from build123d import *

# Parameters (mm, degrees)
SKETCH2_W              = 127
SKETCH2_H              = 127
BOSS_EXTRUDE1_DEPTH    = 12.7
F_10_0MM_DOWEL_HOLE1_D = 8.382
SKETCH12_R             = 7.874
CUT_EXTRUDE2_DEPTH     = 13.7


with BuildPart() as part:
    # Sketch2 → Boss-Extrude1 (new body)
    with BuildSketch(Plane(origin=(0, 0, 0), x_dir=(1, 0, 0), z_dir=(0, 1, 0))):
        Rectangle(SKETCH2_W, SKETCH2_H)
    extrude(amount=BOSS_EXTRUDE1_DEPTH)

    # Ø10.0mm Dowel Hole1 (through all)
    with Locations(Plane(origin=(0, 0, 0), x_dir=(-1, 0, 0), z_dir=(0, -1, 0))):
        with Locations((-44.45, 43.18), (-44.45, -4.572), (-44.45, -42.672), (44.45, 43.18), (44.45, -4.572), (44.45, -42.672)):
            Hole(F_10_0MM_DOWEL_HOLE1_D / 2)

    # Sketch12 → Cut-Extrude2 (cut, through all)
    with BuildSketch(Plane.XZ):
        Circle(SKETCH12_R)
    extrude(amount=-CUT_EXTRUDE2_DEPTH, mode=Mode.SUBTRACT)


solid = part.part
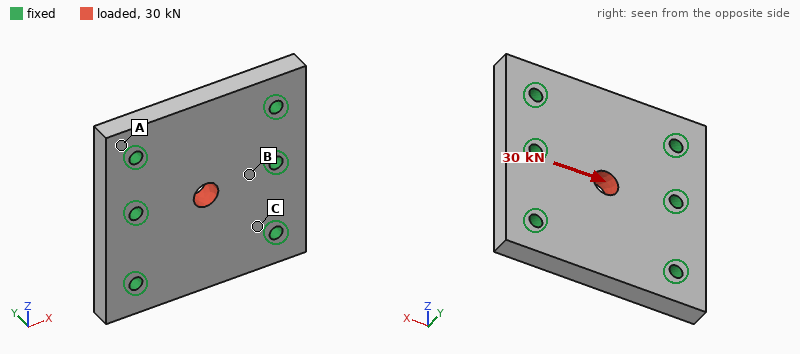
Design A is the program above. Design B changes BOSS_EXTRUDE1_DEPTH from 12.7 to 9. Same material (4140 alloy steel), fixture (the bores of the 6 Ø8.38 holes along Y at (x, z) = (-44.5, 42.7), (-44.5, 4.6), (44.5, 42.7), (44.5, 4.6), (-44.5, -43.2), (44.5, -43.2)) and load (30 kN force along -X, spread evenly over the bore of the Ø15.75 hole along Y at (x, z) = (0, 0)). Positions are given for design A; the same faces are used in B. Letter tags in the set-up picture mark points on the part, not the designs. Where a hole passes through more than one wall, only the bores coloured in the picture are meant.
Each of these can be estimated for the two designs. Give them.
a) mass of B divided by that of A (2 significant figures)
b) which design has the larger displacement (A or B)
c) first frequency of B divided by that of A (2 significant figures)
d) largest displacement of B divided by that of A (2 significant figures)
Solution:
0.71
B
0.77
1.4
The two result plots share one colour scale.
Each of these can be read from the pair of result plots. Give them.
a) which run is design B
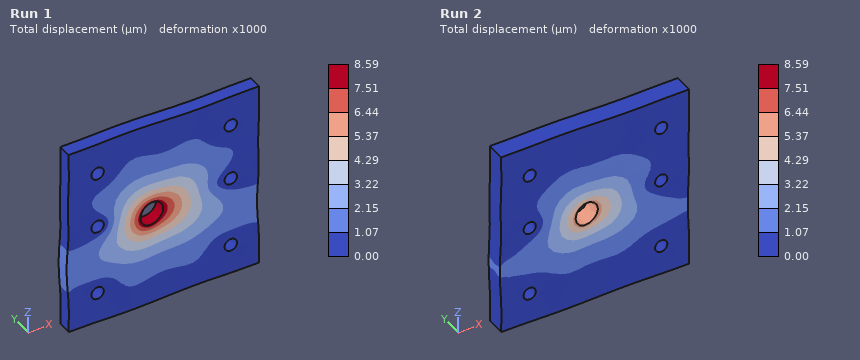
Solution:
Run 1
